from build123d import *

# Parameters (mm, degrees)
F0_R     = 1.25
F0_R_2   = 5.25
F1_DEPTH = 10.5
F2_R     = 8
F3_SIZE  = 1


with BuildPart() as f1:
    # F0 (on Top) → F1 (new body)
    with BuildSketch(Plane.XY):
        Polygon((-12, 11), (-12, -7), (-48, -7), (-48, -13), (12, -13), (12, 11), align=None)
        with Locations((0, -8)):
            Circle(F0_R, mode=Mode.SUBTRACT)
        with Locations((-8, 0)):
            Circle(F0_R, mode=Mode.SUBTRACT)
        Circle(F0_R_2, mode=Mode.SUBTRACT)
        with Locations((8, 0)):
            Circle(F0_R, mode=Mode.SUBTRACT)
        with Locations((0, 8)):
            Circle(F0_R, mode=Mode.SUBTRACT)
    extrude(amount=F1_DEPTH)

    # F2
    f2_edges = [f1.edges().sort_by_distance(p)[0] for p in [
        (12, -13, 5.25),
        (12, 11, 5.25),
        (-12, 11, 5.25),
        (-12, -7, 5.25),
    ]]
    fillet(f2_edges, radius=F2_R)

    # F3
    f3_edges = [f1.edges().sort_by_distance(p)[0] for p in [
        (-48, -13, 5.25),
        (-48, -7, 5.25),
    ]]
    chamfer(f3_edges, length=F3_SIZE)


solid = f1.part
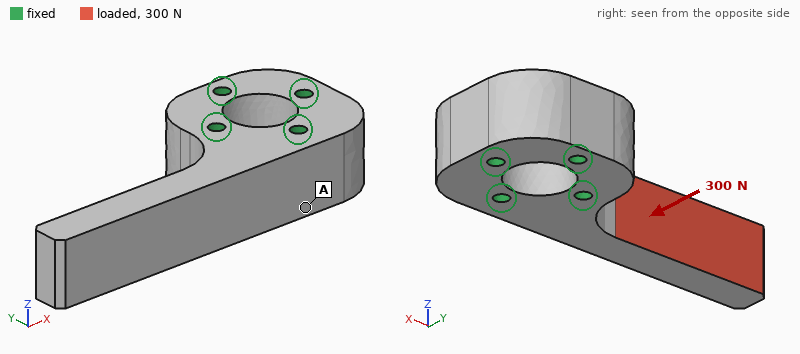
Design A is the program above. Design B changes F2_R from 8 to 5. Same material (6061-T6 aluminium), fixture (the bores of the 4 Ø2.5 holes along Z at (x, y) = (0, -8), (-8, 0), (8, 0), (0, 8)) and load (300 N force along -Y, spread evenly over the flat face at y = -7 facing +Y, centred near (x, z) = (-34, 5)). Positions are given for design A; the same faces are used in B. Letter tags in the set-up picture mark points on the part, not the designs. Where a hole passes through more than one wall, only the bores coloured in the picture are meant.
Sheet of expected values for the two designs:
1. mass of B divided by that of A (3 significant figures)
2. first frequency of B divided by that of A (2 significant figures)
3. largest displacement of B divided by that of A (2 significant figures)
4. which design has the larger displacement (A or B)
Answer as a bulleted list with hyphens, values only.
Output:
- 1.03
- 0.91
- 1.1
- B
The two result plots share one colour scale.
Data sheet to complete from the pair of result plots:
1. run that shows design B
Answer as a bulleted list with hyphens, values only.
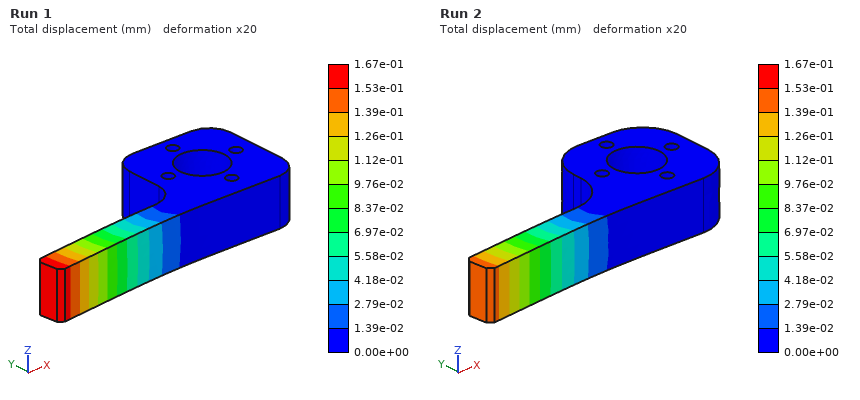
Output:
- Run 1
